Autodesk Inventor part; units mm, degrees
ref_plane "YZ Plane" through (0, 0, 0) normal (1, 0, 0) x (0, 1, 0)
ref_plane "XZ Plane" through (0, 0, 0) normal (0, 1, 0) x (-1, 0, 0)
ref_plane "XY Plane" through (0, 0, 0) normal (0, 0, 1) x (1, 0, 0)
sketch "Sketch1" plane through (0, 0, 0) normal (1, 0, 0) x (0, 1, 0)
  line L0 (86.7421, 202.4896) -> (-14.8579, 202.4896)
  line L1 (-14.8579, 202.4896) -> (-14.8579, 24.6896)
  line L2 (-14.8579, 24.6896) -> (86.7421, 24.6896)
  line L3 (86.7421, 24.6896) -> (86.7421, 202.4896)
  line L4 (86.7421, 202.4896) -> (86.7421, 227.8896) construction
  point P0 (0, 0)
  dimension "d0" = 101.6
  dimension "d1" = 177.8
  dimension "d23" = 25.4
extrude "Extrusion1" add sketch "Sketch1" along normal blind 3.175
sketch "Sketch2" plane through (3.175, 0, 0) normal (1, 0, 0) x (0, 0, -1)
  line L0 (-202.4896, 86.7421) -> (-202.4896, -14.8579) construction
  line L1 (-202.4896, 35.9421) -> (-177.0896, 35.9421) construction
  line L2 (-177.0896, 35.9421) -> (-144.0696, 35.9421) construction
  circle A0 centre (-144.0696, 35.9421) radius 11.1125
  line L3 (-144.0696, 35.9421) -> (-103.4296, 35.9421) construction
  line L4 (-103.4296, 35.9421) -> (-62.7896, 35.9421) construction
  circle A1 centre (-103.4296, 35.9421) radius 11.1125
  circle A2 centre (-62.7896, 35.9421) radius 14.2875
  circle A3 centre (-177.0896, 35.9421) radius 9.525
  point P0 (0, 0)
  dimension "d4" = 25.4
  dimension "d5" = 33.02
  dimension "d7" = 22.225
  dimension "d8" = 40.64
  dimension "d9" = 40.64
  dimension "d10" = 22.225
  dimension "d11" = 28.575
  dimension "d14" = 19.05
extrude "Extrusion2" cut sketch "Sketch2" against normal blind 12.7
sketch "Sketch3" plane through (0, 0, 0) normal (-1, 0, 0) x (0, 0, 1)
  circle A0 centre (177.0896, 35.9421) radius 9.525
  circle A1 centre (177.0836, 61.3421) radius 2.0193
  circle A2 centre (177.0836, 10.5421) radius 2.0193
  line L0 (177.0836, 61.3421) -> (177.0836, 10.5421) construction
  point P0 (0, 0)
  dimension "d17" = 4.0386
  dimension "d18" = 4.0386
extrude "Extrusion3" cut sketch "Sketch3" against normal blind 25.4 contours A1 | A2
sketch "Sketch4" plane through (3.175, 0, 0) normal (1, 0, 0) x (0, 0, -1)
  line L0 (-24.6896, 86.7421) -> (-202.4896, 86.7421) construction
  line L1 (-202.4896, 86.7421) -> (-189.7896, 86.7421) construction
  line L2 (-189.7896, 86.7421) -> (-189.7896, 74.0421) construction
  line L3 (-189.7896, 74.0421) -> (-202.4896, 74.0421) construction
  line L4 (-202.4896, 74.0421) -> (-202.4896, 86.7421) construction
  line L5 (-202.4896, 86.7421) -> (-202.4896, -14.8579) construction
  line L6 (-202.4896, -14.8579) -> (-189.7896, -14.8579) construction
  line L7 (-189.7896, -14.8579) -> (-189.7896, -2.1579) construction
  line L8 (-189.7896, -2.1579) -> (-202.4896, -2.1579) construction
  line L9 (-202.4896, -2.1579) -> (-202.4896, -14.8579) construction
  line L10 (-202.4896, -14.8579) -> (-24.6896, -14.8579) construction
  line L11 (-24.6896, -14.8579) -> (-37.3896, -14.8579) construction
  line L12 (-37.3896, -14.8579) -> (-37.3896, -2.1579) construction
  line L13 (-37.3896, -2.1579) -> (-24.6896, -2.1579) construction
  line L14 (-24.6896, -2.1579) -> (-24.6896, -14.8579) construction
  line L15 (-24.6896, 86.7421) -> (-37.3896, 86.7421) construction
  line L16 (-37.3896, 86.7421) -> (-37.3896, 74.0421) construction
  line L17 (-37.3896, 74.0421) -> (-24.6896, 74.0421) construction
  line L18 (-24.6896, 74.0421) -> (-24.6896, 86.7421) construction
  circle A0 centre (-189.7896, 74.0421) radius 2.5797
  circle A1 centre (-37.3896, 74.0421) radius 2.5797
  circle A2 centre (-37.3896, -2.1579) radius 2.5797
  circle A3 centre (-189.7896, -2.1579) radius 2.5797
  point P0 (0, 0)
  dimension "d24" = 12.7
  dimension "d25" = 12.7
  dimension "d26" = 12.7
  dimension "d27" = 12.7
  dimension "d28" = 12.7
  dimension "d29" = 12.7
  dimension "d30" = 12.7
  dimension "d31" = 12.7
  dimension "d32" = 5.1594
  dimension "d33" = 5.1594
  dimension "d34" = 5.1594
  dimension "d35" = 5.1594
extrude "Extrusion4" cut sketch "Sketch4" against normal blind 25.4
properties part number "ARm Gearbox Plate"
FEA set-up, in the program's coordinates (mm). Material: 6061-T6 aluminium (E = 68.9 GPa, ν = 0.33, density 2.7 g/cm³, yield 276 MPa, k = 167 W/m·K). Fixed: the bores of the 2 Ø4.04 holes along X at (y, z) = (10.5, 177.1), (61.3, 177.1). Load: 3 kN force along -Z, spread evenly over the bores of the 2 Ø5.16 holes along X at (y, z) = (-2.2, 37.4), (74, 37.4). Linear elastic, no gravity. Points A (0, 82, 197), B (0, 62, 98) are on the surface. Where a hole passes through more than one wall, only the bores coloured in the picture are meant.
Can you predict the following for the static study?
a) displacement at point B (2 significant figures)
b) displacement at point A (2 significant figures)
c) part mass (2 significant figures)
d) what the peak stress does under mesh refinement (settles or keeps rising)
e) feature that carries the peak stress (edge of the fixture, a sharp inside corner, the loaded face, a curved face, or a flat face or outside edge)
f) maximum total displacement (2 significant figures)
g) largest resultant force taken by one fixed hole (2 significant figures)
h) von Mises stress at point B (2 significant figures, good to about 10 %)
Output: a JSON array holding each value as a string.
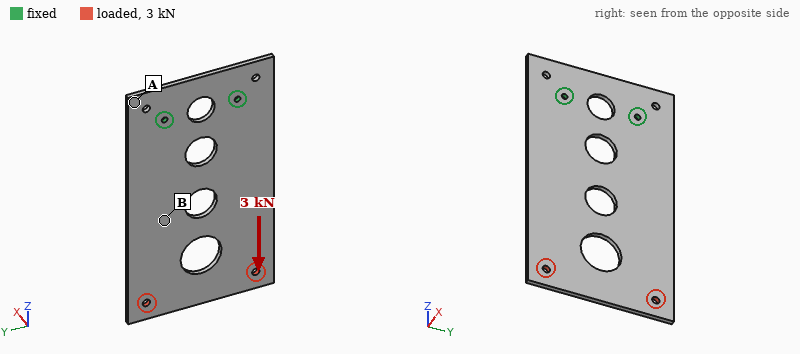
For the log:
["16 µm", "5.9 µm", "140 g", "keeps rising", "edge of the fixture", "32 µm", "1.5 kN", "11 MPa"]
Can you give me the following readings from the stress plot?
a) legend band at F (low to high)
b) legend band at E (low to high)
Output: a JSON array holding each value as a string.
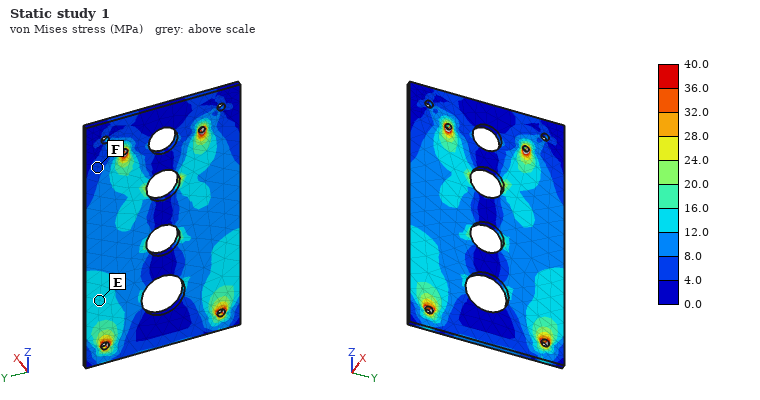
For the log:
["4.0 to 8.0 MPa", "12.0 to 16.0 MPa"]
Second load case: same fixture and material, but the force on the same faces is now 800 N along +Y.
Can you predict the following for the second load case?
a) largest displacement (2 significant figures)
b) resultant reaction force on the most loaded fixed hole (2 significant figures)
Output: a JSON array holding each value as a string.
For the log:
["0.13 mm", "2.1 kN"]
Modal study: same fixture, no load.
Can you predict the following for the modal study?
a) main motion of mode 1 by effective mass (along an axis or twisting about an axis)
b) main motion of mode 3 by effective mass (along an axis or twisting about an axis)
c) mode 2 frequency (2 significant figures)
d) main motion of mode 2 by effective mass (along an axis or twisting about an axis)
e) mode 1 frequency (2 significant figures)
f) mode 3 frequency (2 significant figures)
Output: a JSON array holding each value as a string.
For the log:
["along X", "along X", "340 Hz", "twisting about Z", "110 Hz", "650 Hz"]
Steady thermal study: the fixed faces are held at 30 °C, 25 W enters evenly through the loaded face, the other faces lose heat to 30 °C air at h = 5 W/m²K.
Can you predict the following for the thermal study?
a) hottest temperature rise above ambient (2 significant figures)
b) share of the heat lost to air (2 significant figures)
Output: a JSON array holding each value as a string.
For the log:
["76 K", "23 %"]
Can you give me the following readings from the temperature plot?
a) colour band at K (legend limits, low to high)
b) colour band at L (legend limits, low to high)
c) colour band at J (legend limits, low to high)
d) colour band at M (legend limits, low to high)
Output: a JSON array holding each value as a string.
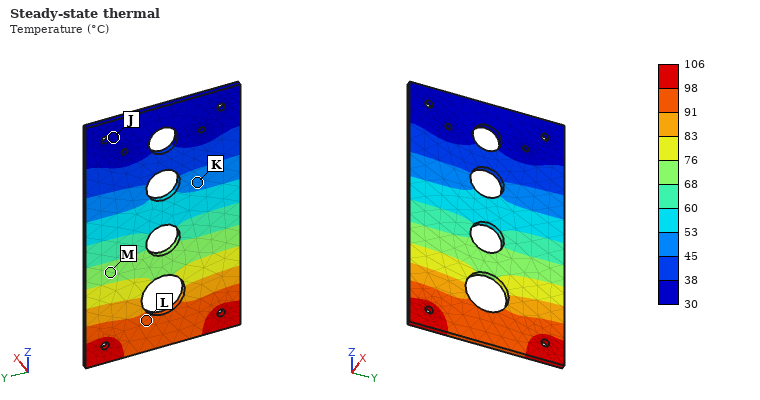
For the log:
["45 to 53 °C", "91 to 98 °C", "30 to 38 °C", "68 to 76 °C"]
